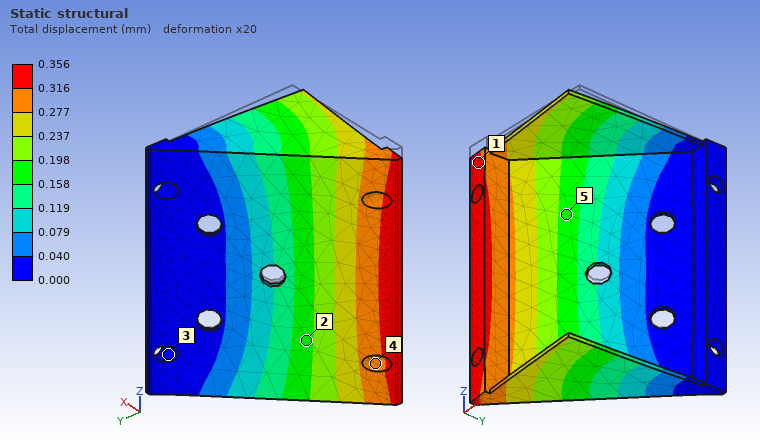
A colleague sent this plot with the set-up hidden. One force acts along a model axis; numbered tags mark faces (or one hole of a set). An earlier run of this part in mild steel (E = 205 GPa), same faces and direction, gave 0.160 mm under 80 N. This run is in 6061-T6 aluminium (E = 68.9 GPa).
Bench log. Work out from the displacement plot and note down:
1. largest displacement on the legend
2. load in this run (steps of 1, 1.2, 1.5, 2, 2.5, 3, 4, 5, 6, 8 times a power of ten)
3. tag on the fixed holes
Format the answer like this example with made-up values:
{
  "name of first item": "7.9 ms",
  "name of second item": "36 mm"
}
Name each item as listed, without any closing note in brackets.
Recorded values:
{
  "largest displacement on the legend": "0.356 mm",
  "load in this run": "60 N",
  "tag on the fixed holes": "3"
}
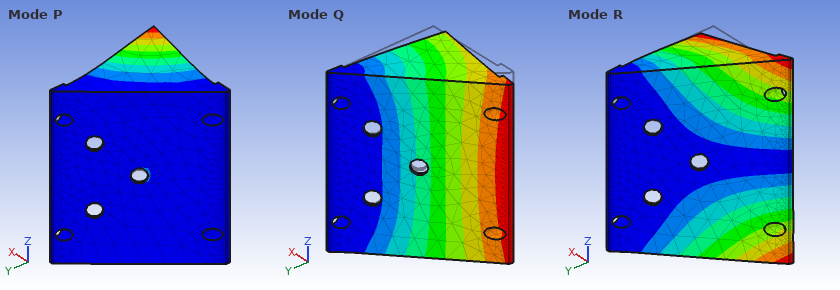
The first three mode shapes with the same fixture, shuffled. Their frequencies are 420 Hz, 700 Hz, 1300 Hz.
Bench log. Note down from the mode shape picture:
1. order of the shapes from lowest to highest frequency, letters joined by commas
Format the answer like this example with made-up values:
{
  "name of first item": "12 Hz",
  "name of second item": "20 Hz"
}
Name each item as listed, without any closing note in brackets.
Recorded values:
{
  "order of the shapes from lowest to highest frequency, letters joined by commas": "Q, R, P"
}
